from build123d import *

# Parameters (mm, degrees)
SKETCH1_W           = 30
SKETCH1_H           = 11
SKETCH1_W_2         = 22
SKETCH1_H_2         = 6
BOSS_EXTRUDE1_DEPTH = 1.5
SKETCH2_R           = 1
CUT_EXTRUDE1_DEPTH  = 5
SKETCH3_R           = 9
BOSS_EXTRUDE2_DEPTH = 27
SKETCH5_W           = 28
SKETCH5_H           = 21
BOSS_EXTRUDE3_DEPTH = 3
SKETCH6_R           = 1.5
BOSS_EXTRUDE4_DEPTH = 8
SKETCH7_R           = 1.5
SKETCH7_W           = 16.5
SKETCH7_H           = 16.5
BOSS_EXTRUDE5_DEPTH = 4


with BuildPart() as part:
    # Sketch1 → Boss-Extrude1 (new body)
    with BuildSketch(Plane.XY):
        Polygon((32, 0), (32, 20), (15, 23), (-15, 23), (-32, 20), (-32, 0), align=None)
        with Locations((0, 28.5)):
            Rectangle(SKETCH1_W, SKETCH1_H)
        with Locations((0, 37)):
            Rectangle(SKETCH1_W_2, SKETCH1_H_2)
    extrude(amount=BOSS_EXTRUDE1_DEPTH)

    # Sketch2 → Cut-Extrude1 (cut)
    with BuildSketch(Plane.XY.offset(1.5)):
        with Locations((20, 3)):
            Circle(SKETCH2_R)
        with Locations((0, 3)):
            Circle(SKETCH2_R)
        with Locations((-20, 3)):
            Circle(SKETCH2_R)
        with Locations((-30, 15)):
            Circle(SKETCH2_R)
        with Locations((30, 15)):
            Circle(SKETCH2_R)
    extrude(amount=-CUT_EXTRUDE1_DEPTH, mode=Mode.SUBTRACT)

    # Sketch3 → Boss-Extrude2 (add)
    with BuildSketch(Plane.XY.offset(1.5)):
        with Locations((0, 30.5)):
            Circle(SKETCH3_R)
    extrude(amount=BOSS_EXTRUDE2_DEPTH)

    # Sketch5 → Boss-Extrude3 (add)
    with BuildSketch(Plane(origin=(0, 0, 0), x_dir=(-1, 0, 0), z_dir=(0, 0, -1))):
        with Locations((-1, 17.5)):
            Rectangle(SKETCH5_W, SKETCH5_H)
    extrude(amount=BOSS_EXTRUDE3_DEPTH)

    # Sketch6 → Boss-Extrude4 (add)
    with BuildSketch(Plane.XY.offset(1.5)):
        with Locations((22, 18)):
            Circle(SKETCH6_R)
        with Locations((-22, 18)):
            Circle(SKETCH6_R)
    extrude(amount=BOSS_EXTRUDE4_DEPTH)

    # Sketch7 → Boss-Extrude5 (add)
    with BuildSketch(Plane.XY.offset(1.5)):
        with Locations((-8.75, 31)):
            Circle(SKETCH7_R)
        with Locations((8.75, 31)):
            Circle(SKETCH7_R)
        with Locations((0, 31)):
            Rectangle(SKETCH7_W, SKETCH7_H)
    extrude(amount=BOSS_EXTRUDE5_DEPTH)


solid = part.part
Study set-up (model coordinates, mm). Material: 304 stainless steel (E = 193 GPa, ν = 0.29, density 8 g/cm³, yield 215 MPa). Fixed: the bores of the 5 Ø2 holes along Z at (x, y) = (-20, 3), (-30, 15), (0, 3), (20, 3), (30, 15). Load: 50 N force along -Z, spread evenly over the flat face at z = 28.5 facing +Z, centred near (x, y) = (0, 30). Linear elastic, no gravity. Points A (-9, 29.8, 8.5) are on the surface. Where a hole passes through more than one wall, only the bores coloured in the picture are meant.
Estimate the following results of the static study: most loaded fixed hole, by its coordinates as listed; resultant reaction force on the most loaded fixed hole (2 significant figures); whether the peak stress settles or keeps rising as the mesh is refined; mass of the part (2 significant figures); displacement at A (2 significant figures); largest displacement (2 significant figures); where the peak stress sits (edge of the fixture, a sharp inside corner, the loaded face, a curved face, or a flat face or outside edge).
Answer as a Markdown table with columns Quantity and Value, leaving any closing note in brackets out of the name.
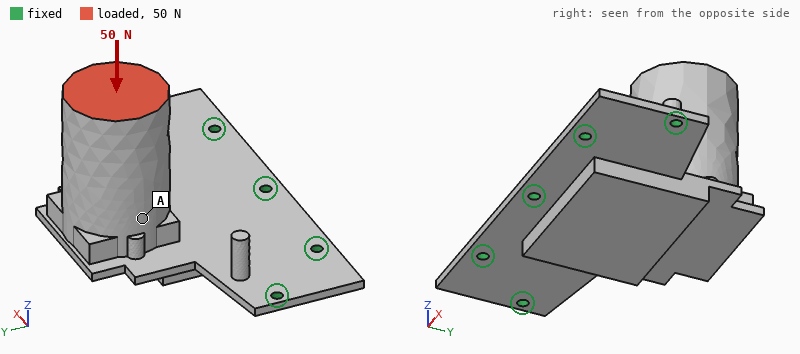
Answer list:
| Quantity | Value |
|---|---|
| most loaded fixed hole, by its coordinates as listed | (30, 15) |
| resultant reaction force on the most loaded fixed hole | 45 N |
| whether the peak stress settles or keeps rising as the mesh is refined | keeps rising |
| mass of the part | 94 g |
| displacement at A | 42 µm |
| largest displacement | 73 µm |
| where the peak stress sits | edge of the fixture |
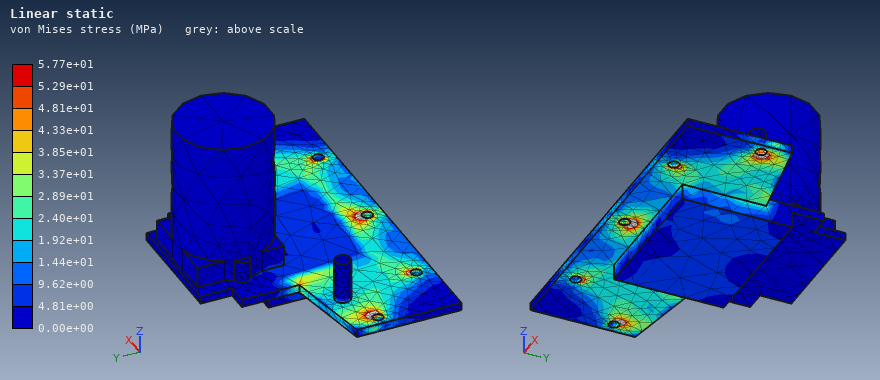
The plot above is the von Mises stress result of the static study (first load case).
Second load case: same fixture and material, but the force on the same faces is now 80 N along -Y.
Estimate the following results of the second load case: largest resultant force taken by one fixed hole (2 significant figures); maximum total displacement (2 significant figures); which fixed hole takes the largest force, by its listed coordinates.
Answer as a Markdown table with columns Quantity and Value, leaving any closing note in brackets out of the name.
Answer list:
| Quantity | Value |
|---|---|
| largest resultant force taken by one fixed hole | 85 N |
| maximum total displacement | 0.14 mm |
| which fixed hole takes the largest force, by its listed coordinates | (30, 15) |
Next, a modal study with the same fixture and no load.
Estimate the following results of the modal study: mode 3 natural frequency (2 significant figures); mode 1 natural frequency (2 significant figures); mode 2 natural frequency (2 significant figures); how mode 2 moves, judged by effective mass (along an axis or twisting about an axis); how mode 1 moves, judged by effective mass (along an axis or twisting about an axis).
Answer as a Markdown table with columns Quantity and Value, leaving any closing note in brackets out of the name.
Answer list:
| Quantity | Value |
|---|---|
| mode 3 natural frequency | 3500 Hz |
| mode 1 natural frequency | 570 Hz |
| mode 2 natural frequency | 1900 Hz |
| how mode 2 moves, judged by effective mass | along X |
| how mode 1 moves, judged by effective mass | along Z |
